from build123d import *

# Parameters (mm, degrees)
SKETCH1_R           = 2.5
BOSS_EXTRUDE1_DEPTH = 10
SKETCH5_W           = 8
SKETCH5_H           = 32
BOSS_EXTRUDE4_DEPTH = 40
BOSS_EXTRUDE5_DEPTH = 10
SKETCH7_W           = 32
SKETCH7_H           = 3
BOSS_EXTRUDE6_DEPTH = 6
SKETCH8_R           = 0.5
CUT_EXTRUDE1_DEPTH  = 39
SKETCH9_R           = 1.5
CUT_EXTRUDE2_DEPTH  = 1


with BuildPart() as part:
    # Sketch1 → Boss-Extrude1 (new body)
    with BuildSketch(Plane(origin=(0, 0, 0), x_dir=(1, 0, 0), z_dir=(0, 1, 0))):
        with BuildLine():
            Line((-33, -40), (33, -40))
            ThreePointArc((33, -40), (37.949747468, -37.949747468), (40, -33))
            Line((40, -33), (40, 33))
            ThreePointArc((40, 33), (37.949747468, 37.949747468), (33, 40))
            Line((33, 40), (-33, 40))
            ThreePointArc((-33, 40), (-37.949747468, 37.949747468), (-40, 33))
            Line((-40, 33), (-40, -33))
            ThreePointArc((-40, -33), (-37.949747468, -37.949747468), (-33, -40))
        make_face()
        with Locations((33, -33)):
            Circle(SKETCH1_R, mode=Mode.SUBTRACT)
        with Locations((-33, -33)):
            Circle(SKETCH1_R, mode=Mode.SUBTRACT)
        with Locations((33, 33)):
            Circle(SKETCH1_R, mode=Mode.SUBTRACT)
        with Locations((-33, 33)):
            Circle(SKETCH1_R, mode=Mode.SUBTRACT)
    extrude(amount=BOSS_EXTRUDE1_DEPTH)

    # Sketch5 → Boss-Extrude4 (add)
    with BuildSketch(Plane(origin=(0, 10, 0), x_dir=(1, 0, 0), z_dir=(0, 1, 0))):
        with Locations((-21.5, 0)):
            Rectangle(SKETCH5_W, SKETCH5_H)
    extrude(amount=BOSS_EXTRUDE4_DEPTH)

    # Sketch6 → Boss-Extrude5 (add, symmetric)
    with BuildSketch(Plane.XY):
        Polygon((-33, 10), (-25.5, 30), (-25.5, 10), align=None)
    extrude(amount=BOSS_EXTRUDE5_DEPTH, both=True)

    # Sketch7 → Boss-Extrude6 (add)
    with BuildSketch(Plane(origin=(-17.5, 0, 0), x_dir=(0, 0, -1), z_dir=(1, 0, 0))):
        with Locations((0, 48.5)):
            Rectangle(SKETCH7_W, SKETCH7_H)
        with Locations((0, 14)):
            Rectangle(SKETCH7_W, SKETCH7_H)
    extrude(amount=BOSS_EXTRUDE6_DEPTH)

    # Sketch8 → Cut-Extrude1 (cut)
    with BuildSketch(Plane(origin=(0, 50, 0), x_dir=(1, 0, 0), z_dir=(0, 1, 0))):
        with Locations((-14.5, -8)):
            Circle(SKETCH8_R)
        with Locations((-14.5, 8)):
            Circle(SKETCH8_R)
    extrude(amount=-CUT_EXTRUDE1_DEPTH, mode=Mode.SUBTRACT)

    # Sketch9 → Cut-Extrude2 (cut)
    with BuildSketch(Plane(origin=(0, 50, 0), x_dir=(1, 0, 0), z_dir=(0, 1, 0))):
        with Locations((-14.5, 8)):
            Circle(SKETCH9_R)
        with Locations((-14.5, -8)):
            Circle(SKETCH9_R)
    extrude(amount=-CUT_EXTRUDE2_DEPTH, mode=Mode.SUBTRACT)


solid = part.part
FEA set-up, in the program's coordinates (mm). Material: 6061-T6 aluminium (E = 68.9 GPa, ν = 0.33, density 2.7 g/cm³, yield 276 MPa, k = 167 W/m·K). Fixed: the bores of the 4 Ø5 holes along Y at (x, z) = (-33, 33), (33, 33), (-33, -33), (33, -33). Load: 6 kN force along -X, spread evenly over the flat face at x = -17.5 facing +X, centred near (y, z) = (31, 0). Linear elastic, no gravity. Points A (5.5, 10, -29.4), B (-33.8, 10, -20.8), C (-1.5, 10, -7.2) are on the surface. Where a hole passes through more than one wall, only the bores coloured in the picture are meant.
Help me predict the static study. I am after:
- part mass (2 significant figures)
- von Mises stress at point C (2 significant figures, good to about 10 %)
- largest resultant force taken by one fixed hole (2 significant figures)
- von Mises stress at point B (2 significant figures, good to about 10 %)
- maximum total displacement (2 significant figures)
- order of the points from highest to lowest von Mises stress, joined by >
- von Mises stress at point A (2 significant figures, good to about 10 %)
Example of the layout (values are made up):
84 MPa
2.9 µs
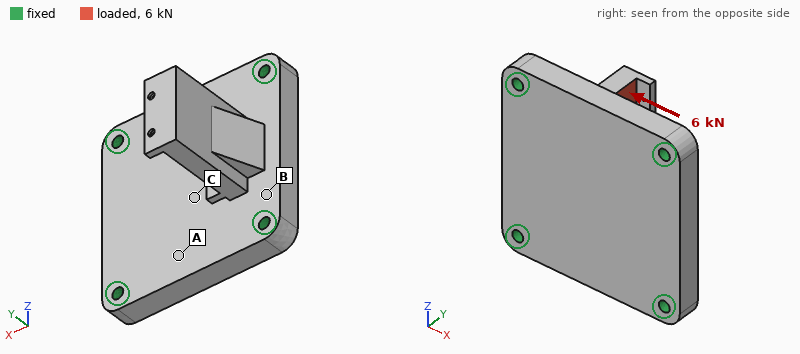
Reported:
200 g
45 MPa
2.2 kN
72 MPa
0.47 mm
B > C > A
22 MPa
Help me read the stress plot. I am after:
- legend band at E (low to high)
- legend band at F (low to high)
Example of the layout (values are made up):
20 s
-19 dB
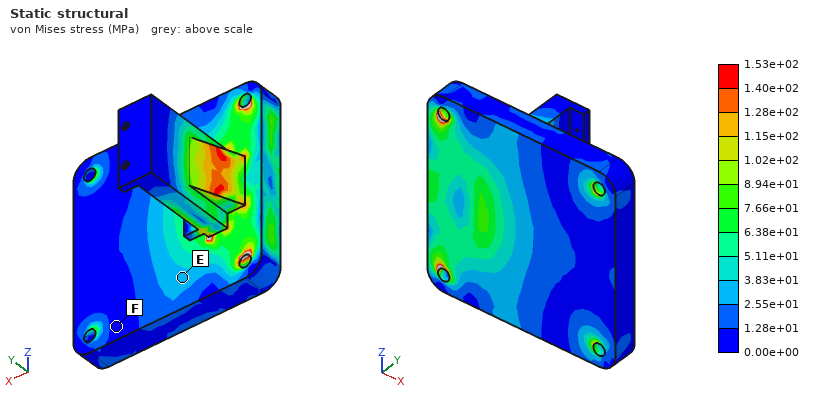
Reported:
2.55e+01 to 3.83e+01 MPa
0.00e+00 to 1.28e+01 MPa
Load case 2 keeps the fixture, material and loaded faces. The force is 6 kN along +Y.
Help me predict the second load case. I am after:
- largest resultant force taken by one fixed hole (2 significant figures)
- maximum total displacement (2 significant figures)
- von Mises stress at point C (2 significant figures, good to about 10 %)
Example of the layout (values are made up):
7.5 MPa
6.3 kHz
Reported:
2.4 kN
0.16 mm
22 MPa
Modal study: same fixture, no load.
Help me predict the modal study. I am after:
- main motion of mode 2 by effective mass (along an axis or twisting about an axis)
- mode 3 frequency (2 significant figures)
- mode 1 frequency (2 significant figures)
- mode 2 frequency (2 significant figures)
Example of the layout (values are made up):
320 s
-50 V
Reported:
along Y
7100 Hz
3900 Hz
6500 Hz
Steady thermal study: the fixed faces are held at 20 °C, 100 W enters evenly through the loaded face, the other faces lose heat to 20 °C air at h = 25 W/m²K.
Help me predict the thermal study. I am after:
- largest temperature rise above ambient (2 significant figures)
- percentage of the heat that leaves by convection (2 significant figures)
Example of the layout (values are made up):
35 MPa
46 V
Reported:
64 K
7.2 %
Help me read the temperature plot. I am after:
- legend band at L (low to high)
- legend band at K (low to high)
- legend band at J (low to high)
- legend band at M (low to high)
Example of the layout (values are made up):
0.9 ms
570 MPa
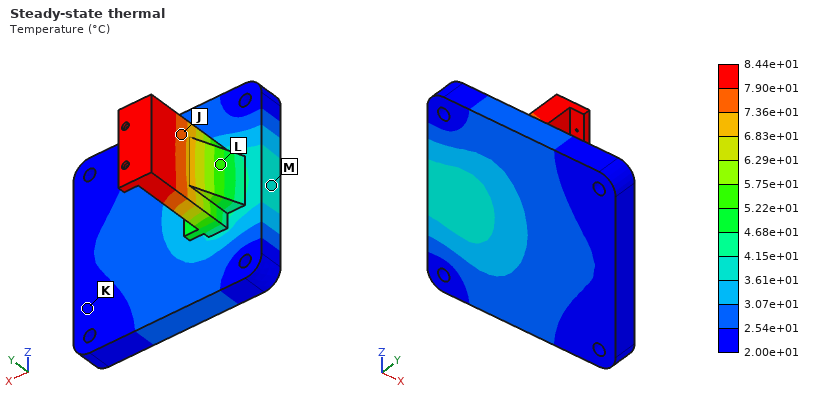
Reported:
5.22e+01 to 5.75e+01 °C
2.00e+01 to 2.54e+01 °C
7.36e+01 to 7.90e+01 °C
3.61e+01 to 4.15e+01 °C
